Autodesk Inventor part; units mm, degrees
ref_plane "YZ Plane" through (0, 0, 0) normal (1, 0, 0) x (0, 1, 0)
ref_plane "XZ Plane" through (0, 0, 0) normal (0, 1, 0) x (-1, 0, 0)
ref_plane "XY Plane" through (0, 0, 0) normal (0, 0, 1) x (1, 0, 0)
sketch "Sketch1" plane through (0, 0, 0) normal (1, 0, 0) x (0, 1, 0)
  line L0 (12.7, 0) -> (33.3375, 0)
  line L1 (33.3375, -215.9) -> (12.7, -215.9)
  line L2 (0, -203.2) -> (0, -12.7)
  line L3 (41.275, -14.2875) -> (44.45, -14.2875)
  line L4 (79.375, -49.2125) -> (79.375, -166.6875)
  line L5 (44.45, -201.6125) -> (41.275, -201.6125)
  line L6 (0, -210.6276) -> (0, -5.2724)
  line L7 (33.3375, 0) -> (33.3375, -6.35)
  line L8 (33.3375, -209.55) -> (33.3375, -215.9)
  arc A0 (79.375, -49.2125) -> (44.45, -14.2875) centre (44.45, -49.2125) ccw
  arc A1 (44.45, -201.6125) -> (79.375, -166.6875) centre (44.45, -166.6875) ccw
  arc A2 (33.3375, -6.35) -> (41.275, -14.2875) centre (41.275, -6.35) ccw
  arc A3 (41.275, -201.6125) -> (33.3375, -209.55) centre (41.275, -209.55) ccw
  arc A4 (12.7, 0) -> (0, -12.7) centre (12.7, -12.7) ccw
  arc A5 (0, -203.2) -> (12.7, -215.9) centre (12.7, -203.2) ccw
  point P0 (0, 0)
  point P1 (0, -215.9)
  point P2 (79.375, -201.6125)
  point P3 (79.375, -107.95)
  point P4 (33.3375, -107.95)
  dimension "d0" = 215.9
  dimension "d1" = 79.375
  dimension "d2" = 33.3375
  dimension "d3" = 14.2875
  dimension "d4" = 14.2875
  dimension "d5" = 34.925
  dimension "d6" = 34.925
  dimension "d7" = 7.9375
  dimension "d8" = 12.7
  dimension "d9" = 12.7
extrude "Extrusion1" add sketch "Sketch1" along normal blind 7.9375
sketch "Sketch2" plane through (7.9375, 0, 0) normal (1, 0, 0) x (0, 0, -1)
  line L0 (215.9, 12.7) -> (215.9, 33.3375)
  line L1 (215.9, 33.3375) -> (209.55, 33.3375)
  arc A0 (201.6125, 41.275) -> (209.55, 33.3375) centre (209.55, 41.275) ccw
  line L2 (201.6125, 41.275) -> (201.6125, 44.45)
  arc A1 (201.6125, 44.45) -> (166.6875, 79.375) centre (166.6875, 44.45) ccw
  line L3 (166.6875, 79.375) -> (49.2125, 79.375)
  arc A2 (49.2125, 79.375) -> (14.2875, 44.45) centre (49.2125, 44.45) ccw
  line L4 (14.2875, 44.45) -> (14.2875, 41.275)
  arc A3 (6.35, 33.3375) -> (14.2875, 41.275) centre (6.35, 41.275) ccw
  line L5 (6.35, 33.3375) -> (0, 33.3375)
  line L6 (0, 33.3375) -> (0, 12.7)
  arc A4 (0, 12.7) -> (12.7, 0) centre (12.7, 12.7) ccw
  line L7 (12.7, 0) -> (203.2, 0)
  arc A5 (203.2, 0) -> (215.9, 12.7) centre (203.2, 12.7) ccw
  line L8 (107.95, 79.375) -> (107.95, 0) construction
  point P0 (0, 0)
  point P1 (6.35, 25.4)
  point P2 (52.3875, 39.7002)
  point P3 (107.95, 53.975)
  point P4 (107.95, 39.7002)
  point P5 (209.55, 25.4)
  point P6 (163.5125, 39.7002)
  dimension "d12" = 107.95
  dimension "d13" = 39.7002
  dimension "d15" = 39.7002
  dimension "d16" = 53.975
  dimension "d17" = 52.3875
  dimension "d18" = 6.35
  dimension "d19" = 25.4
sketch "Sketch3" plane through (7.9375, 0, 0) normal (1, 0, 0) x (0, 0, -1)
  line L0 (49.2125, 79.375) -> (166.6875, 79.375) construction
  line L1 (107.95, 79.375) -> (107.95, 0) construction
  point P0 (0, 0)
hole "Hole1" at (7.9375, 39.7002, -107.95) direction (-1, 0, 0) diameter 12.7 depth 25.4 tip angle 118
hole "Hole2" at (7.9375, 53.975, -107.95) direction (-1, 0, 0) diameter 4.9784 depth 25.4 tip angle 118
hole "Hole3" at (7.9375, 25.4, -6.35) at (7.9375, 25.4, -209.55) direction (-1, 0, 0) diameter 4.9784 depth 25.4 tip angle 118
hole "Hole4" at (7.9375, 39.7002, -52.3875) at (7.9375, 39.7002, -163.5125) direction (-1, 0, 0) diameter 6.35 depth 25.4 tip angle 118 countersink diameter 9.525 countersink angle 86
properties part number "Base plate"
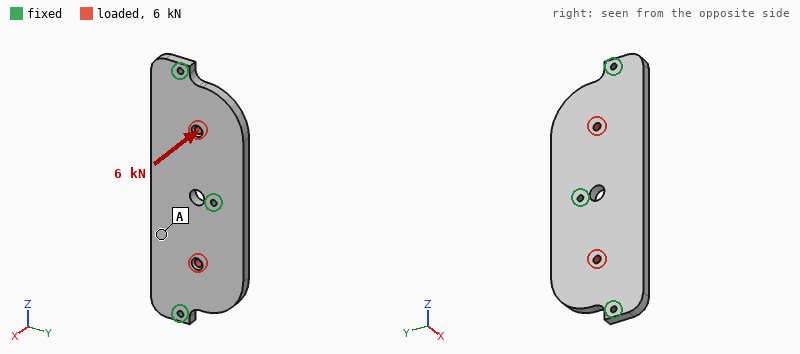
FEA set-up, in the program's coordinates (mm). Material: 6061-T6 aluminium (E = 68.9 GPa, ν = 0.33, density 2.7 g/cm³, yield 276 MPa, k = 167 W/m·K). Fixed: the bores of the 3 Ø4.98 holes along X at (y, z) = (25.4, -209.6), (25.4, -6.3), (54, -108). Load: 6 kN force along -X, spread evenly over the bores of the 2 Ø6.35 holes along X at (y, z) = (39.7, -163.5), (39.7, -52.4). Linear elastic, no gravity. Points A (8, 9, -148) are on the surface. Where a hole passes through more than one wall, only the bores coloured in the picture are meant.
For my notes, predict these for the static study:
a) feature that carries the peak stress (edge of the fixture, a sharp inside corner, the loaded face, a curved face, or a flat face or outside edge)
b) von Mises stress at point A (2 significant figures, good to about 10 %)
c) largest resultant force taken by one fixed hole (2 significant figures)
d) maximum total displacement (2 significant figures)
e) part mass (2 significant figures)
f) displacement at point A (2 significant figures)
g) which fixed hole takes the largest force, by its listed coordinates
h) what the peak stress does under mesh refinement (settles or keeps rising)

edge of the fixture
29 MPa
3.0 kN
0.15 mm
320 g
0.12 mm
(54, -108)
keeps rising
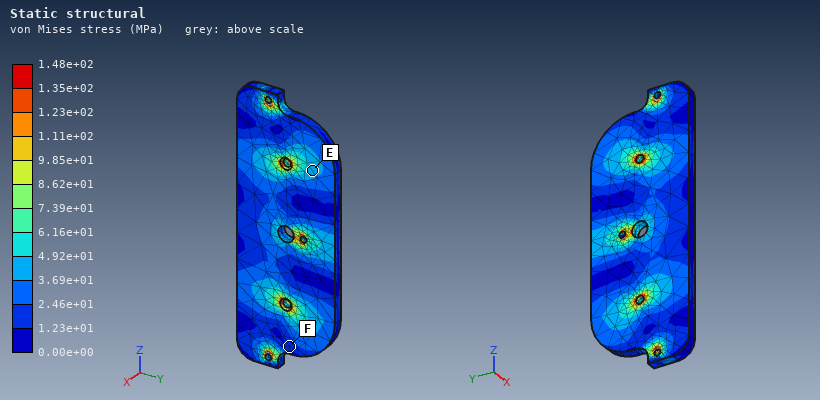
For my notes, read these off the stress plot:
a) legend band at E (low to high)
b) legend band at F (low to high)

3.69e+01 to 4.92e+01 MPa
1.23e+01 to 2.46e+01 MPa
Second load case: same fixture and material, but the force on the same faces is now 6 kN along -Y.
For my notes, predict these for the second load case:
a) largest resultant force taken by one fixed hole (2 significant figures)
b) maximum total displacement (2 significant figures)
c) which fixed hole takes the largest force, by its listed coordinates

3.4 kN
16 µm
(54, -108)
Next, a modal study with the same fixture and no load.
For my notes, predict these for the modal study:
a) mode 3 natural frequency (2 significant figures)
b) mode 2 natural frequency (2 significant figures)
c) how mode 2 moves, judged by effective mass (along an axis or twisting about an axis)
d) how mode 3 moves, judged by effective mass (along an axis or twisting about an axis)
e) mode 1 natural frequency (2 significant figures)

2500 Hz
2200 Hz
twisting about Y
along X
1700 Hz
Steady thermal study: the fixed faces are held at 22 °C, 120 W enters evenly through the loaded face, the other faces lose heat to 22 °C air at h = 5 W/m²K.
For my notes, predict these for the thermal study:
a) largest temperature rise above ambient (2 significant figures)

39 K
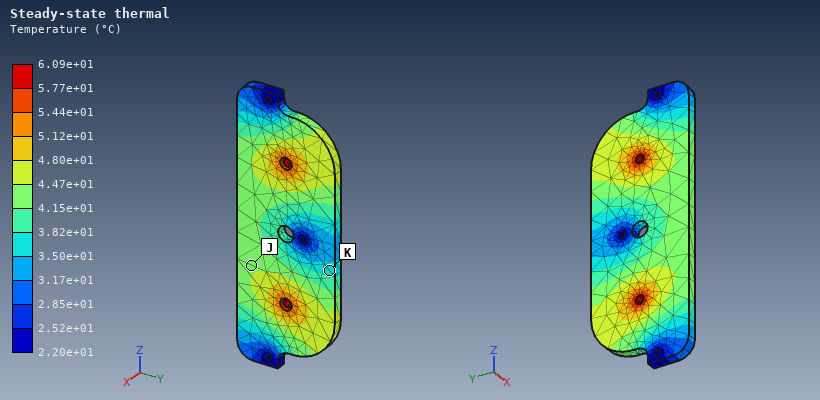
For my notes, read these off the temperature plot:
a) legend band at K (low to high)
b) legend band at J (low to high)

3.50e+01 to 3.82e+01 °C
4.15e+01 to 4.47e+01 °C
